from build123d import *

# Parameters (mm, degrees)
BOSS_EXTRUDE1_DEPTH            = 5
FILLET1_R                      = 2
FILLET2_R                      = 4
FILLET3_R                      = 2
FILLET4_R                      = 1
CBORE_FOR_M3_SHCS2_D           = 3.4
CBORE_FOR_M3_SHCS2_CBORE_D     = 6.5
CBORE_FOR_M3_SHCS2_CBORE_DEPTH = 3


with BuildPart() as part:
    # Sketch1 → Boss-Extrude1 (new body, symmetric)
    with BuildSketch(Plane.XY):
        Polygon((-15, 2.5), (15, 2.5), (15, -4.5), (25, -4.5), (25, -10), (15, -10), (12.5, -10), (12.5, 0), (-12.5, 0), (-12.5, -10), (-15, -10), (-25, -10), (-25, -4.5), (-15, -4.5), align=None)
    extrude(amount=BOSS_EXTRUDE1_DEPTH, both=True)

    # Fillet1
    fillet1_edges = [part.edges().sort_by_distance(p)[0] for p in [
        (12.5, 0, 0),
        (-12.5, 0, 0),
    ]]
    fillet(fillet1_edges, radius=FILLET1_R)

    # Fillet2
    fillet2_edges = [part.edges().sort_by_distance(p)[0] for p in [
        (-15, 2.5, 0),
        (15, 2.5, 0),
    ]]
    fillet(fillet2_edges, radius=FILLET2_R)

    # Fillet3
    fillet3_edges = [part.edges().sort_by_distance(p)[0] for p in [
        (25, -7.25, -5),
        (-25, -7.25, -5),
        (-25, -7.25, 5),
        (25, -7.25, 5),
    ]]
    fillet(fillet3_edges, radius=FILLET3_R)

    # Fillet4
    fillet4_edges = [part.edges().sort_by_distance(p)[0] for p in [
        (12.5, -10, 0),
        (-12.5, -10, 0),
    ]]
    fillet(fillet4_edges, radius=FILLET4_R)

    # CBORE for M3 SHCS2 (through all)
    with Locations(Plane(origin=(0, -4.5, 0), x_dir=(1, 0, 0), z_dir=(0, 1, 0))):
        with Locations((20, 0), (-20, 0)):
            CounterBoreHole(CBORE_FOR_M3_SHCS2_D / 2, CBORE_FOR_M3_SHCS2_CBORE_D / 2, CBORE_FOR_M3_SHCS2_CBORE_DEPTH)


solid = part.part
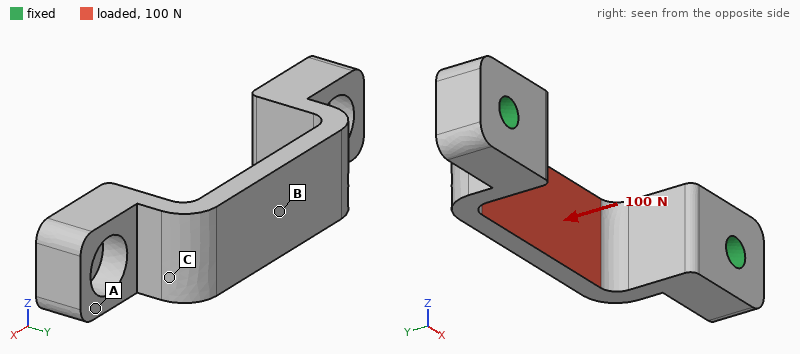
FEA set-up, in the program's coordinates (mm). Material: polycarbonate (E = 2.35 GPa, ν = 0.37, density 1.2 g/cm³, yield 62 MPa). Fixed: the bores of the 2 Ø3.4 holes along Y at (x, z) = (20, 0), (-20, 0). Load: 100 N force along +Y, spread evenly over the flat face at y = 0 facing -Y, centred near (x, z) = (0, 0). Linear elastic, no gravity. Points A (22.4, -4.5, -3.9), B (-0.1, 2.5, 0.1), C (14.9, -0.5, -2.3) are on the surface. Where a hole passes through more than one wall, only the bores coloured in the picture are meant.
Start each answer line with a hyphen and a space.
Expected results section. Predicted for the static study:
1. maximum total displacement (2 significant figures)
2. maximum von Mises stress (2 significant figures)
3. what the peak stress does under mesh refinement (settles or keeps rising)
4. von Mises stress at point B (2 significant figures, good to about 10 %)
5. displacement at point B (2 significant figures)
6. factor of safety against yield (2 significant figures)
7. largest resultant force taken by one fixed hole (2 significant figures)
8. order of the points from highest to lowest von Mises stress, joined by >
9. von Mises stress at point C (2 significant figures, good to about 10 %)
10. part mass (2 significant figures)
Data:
- 0.27 mm
- 23 MPa
- settles
- 16 MPa
- 0.25 mm
- 2.7
- 72 N
- B > C > A
- 7.4 MPa
- 2.4 g
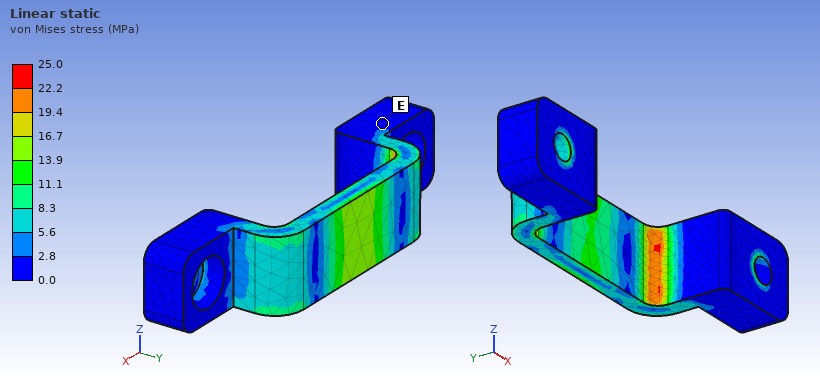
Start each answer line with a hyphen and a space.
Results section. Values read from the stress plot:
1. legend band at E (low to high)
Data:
- 0.0 to 2.8 MPa
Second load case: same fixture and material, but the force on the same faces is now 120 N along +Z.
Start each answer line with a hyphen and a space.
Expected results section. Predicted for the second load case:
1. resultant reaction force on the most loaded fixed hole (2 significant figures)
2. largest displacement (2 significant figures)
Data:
- 60 N
- 0.34 mm
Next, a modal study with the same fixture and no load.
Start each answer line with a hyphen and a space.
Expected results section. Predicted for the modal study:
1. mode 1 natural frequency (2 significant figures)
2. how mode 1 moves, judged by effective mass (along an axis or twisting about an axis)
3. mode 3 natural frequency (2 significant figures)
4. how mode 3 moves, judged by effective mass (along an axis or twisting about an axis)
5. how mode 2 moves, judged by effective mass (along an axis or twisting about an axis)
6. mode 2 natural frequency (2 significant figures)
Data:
- 3000 Hz
- along Z
- 4400 Hz
- along Y
- along X
- 3500 Hz
